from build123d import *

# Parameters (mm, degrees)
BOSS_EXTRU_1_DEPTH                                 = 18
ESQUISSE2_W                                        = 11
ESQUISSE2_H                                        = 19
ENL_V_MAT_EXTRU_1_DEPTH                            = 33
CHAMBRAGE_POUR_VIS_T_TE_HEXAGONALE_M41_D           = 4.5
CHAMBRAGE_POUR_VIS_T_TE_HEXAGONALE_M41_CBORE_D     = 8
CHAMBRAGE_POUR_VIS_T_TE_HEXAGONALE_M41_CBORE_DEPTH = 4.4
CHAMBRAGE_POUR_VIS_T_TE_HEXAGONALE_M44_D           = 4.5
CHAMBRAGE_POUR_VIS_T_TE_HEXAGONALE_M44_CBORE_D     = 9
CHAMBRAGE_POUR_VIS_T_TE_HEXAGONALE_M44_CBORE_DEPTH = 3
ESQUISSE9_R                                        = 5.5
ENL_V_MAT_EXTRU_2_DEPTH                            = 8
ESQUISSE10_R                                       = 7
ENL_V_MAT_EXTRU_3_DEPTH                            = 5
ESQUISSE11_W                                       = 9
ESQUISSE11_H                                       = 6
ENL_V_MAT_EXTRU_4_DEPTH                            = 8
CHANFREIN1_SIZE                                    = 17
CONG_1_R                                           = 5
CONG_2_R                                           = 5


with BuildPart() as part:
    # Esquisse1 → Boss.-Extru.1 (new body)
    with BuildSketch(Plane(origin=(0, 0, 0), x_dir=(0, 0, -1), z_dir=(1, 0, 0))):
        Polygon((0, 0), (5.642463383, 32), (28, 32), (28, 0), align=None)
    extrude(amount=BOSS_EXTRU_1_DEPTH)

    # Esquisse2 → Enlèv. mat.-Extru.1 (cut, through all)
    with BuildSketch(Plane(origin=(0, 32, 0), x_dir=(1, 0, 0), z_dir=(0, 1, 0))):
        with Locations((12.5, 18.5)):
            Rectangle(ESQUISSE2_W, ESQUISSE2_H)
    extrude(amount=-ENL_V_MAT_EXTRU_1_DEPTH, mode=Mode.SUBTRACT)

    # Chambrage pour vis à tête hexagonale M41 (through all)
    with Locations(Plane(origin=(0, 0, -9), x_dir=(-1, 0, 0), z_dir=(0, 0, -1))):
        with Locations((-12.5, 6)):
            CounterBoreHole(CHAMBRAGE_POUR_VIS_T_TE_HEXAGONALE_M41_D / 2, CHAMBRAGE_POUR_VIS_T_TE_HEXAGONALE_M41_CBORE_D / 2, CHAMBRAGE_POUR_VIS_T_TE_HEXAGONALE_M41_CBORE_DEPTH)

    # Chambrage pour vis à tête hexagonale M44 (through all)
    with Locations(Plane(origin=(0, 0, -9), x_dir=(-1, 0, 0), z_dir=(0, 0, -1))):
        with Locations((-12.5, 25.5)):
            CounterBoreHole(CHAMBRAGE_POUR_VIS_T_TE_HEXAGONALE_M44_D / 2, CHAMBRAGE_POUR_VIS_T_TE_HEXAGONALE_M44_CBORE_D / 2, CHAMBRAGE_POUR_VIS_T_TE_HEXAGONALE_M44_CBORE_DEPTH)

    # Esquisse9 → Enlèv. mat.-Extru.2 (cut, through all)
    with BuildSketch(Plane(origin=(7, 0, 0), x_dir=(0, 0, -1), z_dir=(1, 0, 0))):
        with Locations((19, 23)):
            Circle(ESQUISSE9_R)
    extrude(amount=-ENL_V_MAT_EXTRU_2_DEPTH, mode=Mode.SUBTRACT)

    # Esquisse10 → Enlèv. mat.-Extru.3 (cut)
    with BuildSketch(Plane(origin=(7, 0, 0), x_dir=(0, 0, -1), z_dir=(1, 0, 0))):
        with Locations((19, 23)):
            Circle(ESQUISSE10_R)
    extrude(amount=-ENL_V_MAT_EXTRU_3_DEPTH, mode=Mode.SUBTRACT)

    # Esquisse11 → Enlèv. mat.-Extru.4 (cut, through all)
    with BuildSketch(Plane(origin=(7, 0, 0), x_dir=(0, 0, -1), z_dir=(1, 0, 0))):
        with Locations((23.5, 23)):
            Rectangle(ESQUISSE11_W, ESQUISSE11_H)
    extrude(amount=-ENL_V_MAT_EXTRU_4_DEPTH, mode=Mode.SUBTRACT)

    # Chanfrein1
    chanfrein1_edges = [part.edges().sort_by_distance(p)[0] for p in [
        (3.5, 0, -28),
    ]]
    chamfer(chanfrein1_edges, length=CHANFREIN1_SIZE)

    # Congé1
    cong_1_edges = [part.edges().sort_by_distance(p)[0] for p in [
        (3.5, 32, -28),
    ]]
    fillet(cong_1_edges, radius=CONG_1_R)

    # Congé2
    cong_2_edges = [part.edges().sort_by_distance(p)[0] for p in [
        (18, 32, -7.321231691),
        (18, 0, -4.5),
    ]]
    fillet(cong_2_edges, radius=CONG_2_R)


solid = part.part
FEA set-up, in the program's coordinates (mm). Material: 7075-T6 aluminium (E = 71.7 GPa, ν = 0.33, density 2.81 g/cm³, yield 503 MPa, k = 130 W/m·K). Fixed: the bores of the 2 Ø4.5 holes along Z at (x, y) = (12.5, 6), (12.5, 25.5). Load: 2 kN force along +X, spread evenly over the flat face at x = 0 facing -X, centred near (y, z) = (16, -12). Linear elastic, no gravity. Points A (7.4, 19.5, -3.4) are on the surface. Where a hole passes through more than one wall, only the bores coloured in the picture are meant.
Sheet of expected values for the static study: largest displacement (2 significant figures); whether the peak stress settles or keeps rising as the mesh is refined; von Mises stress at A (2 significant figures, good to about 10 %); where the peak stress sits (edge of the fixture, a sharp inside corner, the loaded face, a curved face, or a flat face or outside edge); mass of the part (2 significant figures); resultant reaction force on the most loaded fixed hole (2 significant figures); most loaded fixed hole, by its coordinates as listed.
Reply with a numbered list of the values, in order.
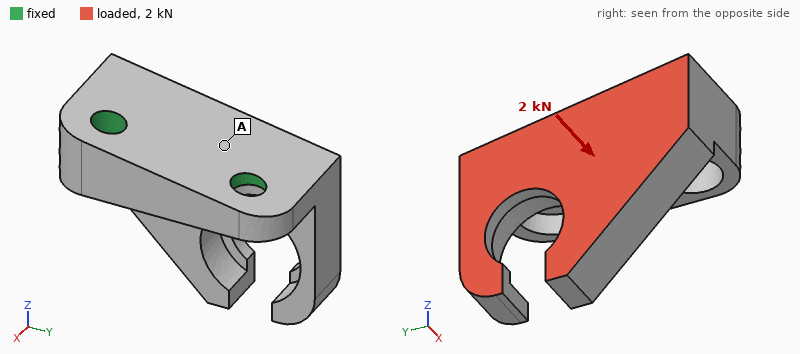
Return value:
1. 0.28 mm
2. keeps rising
3. 79 MPa
4. edge of the fixture
5. 14 g
6. 1.1 kN
7. (12.5, 25.5)
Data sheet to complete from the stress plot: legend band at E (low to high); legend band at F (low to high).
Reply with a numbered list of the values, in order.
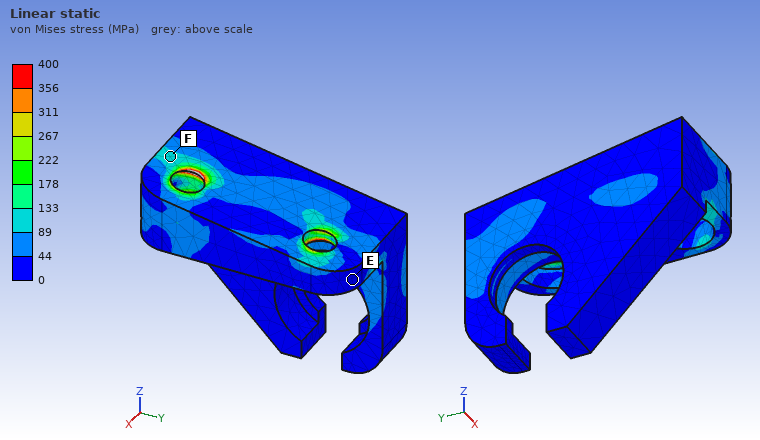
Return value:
1. 0 to 44 MPa
2. 89 to 133 MPa
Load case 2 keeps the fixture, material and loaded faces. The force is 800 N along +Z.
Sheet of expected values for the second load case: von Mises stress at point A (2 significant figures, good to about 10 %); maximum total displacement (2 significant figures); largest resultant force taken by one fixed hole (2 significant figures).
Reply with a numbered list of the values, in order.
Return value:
1. 36 MPa
2. 0.12 mm
3. 430 N
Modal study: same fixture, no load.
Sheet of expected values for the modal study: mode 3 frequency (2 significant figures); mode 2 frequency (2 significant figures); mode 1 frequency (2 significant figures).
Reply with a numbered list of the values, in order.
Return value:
1. 11 kHz
2. 8500 Hz
3. 5600 Hz
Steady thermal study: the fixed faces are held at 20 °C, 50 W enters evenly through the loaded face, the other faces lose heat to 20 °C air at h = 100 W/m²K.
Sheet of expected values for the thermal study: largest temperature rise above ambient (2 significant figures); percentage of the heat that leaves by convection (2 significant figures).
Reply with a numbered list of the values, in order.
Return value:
1. 47 K
2. 10 %
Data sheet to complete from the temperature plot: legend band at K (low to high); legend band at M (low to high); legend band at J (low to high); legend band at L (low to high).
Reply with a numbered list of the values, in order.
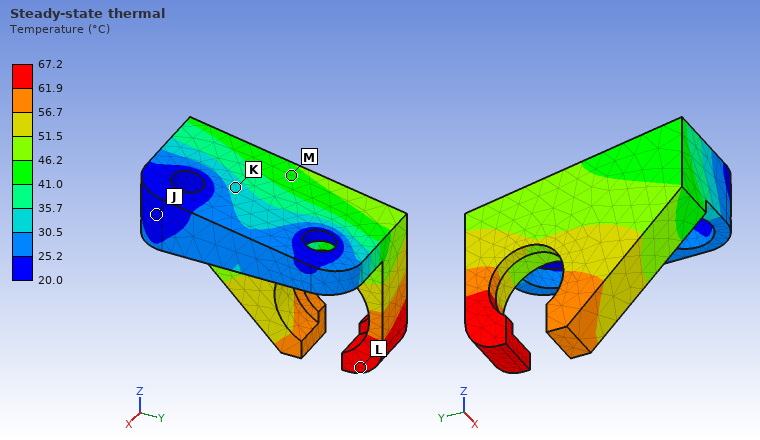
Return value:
1. 30.5 to 35.7 °C
2. 41.0 to 46.2 °C
3. 20.0 to 25.2 °C
4. 61.9 to 67.2 °C
